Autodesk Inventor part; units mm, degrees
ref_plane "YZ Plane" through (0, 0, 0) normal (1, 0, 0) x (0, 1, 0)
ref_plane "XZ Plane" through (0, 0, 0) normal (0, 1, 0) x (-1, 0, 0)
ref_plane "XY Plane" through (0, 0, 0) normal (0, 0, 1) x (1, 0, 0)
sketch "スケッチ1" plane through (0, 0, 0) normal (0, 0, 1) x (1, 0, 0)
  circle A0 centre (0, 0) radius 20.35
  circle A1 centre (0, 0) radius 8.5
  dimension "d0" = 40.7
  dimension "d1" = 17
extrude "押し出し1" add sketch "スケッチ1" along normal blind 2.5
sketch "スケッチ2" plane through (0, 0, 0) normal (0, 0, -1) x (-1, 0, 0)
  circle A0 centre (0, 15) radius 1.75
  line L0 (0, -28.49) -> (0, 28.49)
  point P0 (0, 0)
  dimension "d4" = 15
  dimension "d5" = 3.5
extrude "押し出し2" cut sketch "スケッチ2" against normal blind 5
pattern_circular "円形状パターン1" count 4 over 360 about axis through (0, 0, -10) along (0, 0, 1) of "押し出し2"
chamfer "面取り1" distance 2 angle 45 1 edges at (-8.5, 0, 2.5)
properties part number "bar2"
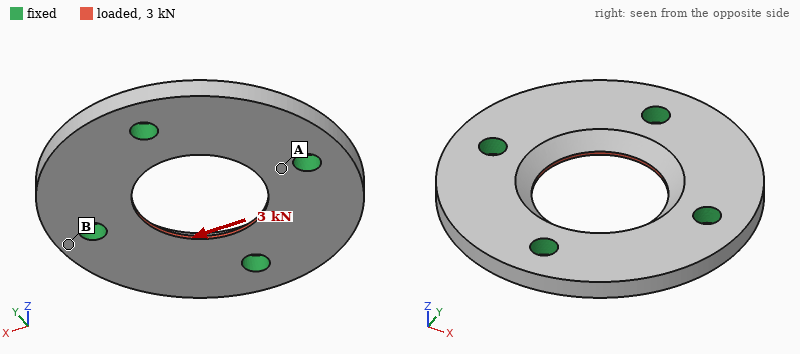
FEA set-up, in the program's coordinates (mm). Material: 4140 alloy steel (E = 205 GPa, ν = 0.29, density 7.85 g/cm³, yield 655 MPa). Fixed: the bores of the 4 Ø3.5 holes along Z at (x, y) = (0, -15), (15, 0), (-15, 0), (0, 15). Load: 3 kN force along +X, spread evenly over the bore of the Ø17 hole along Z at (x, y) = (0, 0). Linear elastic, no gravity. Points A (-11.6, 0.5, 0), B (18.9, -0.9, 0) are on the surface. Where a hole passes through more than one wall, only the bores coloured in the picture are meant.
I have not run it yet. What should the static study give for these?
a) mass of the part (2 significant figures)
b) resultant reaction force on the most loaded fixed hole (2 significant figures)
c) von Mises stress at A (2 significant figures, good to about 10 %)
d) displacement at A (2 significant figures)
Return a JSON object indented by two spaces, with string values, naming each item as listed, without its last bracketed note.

{
  "mass of the part": "19 g",
  "resultant reaction force on the most loaded fixed hole": "770 N",
  "von Mises stress at A": "83 MPa",
  "displacement at A": "0.82 µm"
}
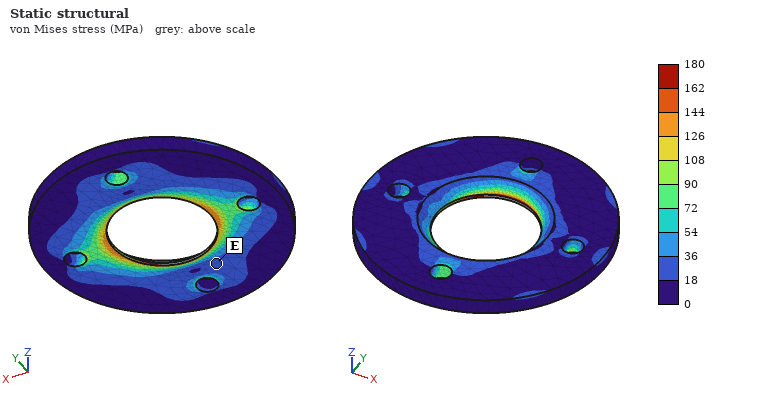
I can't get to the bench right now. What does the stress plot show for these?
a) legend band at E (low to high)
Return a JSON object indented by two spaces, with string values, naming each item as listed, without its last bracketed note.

{
  "legend band at E": "18 to 36 MPa"
}
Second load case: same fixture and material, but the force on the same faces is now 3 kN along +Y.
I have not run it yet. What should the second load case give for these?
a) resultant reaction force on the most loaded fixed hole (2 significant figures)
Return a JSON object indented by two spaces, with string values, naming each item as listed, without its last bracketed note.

{
  "resultant reaction force on the most loaded fixed hole": "770 N"
}
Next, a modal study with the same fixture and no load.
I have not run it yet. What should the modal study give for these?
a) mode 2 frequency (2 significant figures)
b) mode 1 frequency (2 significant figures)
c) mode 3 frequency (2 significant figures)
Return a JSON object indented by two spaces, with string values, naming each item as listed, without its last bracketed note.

{
  "mode 2 frequency": "20 kHz",
  "mode 1 frequency": "20 kHz",
  "mode 3 frequency": "20 kHz"
}
